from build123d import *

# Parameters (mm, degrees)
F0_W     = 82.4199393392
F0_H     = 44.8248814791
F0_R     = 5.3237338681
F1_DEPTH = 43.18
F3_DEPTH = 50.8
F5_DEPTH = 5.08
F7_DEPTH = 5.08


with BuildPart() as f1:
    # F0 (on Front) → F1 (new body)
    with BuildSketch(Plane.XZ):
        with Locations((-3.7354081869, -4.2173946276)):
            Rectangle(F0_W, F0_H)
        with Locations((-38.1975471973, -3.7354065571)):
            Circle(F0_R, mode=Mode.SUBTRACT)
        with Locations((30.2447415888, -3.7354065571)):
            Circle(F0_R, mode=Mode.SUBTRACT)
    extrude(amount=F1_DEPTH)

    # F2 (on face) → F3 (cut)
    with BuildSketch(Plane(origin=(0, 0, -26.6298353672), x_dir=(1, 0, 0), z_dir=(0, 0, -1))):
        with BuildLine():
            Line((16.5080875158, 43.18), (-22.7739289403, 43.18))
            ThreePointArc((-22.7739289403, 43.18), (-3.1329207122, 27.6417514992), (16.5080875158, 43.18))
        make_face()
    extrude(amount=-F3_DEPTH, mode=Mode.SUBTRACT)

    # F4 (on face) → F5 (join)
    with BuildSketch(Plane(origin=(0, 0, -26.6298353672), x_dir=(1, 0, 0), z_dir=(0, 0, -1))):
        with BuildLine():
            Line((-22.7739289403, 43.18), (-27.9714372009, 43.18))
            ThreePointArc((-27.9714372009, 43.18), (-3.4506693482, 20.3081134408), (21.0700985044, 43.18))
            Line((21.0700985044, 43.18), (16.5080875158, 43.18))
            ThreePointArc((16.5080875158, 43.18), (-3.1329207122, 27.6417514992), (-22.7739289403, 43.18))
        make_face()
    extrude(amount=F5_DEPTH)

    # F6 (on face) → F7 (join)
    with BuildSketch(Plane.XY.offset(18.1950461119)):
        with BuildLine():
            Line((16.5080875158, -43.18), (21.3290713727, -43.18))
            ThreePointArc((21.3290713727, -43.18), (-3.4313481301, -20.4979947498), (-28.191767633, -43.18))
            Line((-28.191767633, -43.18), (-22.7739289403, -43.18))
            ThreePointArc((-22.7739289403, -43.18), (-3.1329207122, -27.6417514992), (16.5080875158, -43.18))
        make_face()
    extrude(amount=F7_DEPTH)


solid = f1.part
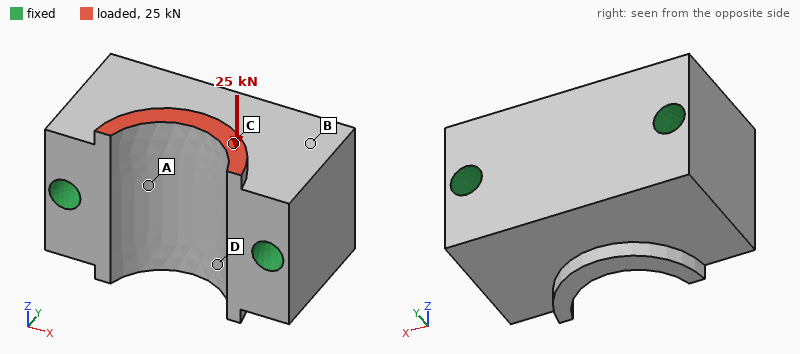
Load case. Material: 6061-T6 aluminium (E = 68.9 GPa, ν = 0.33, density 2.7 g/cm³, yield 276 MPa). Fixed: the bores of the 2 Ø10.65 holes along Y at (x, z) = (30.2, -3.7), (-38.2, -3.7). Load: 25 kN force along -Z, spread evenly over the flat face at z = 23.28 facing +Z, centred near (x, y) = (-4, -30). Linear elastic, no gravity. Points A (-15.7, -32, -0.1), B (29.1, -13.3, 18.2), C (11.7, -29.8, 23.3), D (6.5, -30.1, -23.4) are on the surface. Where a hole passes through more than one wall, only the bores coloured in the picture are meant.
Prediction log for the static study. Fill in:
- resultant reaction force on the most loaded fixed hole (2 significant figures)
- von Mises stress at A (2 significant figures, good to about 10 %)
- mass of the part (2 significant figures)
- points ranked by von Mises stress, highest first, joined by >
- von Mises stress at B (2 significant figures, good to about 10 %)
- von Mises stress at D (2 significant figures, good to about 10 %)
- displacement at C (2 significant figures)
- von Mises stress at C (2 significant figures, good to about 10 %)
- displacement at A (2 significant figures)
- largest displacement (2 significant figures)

13 kN
22 MPa
370 g
C > A > D > B
6.1 MPa
13 MPa
23 µm
55 MPa
10 µm
33 µm
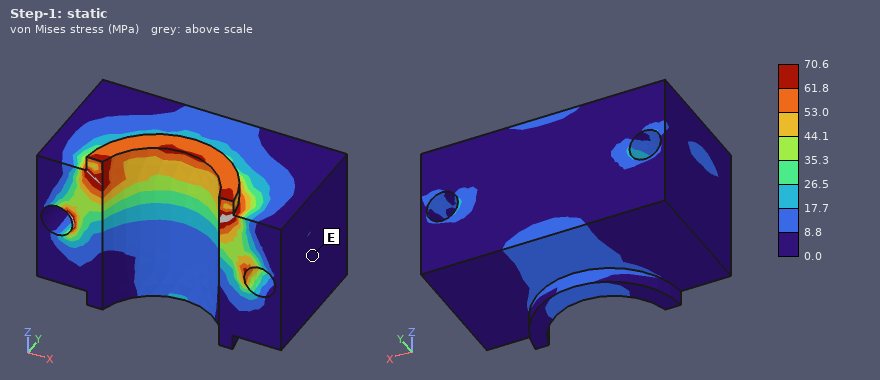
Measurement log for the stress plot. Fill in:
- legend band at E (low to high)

0.0 to 8.8 MPa
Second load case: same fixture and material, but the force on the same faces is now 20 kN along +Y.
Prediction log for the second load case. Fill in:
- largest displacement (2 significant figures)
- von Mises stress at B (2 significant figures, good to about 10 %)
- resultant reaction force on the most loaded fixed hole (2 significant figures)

71 µm
15 MPa
10 kN
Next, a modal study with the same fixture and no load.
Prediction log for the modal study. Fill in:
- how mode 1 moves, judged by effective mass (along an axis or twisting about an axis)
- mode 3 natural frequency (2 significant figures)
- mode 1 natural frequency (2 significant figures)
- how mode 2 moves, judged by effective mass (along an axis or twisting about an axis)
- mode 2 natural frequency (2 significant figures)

along Z
22 kHz
17 kHz
along Y
18 kHz
